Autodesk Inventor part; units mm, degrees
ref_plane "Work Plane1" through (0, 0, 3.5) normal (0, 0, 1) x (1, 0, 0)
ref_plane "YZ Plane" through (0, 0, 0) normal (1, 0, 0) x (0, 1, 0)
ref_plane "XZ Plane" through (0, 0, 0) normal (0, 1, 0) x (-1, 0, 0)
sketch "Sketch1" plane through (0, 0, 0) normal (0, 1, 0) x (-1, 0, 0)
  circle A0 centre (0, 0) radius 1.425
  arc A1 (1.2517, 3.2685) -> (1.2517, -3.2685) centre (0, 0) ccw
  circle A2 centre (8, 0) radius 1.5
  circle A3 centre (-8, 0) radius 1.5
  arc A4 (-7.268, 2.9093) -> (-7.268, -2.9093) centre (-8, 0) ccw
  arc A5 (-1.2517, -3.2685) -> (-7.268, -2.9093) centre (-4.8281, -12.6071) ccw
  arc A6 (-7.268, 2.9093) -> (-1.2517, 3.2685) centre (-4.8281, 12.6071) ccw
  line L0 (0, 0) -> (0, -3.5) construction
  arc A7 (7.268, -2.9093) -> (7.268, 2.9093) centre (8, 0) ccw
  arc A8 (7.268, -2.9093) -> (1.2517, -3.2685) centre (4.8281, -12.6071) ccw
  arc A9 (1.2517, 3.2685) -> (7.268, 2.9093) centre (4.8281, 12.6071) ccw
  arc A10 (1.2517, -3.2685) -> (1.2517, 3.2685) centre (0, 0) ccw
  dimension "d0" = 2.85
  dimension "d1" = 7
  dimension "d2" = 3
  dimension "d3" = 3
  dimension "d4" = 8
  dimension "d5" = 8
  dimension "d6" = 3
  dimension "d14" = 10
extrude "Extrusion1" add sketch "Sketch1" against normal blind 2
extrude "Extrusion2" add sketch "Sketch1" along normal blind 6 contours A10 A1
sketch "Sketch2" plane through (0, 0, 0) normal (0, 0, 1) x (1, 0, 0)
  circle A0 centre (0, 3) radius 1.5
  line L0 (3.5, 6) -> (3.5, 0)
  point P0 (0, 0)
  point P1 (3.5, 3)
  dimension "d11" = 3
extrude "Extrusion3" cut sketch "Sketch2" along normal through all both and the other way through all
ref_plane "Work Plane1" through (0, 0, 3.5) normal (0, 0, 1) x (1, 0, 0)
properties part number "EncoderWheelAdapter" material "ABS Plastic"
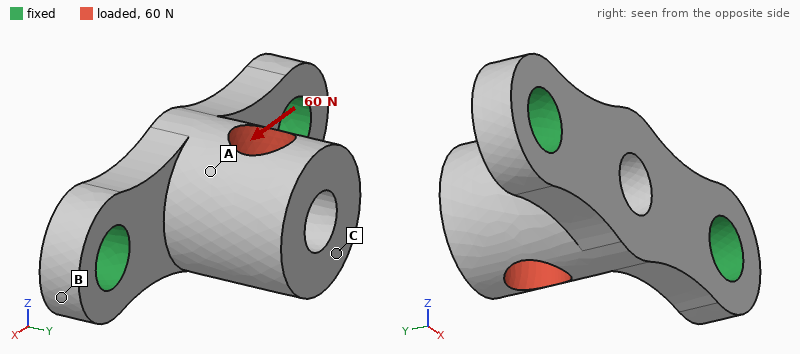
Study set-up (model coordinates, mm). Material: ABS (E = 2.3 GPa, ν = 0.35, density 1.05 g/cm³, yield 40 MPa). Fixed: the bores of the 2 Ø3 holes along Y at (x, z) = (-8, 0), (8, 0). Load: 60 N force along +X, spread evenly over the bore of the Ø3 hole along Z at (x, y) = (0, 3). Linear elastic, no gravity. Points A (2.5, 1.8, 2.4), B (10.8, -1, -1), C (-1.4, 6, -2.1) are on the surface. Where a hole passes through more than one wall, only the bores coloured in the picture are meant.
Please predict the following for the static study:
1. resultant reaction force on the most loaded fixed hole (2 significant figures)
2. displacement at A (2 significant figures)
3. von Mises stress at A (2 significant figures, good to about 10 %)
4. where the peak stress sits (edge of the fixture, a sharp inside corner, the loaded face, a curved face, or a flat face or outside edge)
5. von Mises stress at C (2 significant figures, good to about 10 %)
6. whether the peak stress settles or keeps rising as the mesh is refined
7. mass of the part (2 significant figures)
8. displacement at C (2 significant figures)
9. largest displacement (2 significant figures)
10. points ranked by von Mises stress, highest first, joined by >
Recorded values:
38 N
35 µm
5.1 MPa
edge of the fixture
3.3 MPa
keeps rising
0.38 g
76 µm
83 µm
A > C > B
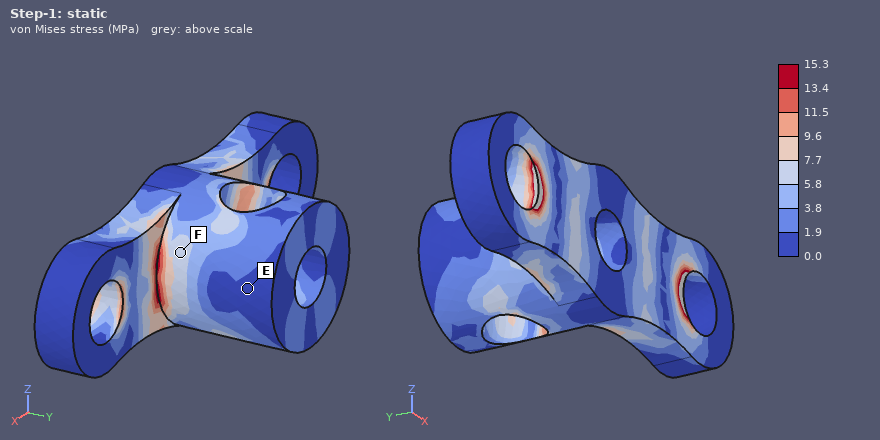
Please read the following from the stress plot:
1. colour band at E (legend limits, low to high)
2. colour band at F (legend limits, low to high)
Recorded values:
0.0 to 1.9 MPa
5.8 to 7.7 MPa
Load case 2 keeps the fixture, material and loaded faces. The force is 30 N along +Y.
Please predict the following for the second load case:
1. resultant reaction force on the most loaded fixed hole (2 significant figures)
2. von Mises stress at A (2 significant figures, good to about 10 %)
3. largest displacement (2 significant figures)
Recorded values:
17 N
1.4 MPa
28 µm
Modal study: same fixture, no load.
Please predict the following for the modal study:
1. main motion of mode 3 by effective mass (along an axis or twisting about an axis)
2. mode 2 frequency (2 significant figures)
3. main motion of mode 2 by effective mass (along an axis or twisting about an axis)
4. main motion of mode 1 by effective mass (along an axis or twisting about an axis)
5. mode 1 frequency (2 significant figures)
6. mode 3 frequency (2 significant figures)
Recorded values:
along X
11 kHz
along Y
along Z
5400 Hz
12 kHz
